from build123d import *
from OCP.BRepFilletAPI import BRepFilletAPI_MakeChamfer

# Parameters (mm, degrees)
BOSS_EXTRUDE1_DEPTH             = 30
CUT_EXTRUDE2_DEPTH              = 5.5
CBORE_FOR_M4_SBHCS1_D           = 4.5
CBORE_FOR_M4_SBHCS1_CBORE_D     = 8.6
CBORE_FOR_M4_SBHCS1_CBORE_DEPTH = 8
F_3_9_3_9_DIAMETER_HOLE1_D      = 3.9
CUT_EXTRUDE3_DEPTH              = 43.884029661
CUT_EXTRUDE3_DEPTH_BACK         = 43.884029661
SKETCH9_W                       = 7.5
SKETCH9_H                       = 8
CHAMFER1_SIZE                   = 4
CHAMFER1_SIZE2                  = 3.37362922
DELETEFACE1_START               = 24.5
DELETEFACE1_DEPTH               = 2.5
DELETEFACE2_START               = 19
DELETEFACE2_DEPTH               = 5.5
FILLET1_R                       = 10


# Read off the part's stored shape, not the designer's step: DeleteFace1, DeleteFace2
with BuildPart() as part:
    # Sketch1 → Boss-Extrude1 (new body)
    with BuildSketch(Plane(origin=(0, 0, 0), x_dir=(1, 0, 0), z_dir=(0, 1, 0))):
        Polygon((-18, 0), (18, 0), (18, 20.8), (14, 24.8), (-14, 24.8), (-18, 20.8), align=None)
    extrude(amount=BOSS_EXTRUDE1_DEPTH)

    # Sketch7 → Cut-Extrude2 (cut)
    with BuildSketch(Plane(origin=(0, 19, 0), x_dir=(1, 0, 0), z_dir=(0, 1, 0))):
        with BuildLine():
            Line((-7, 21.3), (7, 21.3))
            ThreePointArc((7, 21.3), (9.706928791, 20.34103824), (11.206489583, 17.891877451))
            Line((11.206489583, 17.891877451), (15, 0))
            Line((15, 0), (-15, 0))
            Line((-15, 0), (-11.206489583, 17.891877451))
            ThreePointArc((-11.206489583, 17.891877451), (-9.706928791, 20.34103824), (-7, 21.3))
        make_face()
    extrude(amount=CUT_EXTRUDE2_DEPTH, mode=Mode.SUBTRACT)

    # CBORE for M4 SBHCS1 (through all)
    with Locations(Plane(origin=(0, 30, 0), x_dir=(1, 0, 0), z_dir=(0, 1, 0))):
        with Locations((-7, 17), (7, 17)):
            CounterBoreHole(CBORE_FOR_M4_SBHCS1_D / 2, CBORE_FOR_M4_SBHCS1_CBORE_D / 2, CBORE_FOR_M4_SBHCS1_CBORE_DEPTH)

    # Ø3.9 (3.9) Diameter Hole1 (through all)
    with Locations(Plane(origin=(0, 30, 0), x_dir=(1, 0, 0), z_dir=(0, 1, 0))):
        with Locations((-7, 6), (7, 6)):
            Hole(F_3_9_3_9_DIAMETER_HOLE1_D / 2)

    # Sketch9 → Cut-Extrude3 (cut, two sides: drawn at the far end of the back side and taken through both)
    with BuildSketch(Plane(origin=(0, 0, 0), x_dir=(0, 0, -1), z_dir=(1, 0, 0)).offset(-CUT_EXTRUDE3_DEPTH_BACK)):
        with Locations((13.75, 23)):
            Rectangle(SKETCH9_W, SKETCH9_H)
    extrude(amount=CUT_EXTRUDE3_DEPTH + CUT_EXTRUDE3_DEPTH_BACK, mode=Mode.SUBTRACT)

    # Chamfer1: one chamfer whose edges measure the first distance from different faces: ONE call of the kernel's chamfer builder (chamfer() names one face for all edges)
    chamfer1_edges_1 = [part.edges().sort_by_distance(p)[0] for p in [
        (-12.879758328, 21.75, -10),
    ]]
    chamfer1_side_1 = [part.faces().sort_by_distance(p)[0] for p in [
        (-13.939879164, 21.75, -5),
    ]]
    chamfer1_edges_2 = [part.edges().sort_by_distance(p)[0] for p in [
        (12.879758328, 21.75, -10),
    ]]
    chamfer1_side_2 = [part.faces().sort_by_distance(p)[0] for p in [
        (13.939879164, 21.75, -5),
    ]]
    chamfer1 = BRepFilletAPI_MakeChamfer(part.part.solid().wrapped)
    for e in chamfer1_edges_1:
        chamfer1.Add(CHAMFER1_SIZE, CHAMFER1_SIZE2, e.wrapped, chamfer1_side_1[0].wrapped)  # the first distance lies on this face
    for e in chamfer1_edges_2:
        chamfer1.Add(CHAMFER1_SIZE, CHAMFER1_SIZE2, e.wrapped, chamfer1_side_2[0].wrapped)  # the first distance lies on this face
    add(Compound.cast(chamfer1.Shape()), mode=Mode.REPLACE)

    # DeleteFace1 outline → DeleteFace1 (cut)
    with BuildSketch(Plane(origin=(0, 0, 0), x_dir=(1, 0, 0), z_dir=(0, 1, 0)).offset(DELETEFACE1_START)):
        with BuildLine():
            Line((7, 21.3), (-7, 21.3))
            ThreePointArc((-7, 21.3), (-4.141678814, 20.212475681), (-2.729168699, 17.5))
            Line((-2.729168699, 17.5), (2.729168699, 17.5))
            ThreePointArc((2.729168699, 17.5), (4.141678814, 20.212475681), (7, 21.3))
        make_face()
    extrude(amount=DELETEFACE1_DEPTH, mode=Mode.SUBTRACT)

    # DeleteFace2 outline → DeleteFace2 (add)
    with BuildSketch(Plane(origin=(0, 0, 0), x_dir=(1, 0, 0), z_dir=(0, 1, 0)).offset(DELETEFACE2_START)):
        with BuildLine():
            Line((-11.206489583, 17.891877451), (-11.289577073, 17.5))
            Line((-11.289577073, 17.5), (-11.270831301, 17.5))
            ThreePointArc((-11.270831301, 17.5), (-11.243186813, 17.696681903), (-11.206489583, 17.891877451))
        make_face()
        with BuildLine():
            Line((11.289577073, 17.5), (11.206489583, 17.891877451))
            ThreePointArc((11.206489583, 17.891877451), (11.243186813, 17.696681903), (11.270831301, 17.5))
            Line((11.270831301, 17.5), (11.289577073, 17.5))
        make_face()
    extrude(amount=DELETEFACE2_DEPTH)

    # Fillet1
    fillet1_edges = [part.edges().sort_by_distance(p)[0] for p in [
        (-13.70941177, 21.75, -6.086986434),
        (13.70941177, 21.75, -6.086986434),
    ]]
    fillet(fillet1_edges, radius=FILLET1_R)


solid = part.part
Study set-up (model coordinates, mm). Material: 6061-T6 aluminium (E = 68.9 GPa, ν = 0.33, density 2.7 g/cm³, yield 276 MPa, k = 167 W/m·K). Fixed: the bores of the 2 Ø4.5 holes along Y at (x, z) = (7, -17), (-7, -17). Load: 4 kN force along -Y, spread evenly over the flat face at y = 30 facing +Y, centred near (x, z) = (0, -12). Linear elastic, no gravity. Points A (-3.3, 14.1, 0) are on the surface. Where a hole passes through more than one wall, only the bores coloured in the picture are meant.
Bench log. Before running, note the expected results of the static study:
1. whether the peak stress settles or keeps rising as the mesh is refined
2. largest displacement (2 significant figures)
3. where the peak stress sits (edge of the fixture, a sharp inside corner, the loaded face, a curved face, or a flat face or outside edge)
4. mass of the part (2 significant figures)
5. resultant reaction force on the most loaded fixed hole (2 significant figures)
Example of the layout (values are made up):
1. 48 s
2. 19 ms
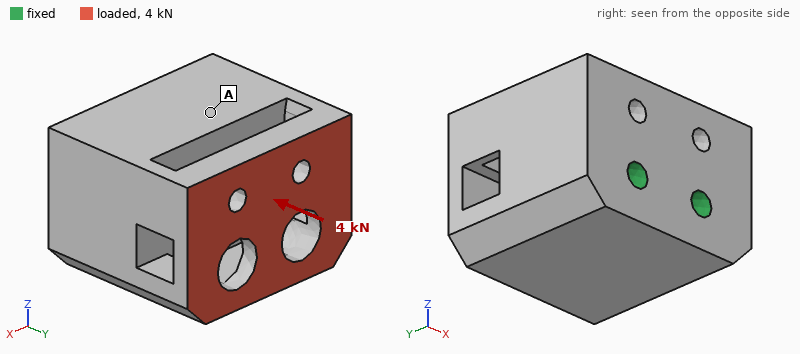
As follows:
1. keeps rising
2. 61 µm
3. a sharp inside corner
4. 55 g
5. 2.0 kN
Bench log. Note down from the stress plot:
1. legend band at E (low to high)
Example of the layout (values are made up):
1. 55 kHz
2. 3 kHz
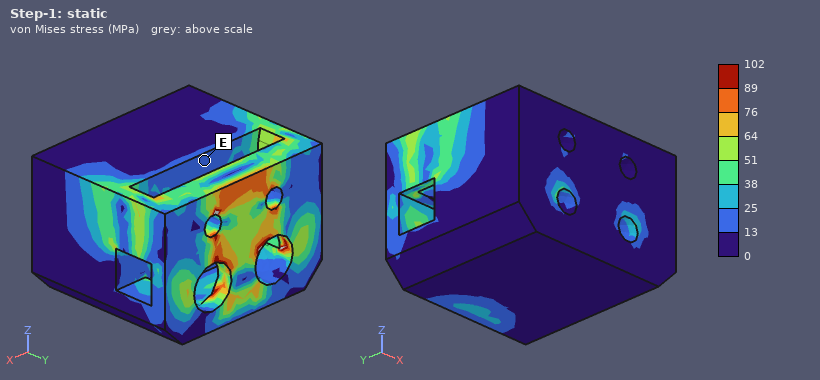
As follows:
1. 13 to 25 MPa
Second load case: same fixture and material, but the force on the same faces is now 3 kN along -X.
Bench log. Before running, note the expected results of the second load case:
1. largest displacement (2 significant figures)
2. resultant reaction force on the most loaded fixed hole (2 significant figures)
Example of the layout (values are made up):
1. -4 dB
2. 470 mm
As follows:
1. 44 µm
2. 2.4 kN
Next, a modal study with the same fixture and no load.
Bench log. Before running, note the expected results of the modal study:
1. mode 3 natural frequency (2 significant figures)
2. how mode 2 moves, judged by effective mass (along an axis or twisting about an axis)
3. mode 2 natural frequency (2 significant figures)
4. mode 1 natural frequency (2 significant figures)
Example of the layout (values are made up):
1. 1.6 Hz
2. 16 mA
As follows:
1. 17 kHz
2. along X
3. 15 kHz
4. 14 kHz
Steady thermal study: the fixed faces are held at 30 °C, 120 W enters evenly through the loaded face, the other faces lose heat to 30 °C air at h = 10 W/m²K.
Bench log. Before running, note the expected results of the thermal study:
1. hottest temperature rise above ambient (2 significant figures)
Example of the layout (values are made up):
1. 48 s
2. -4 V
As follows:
1. 75 K
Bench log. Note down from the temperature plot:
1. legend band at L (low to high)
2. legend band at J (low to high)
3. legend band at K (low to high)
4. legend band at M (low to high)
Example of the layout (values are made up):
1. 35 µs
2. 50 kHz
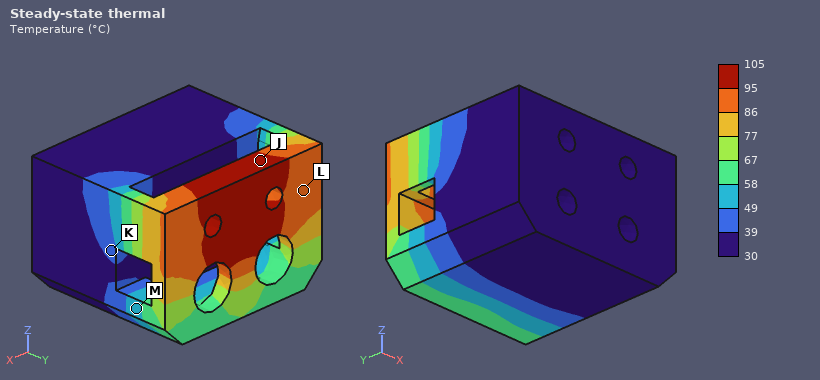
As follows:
1. 86 to 95 °C
2. 95 to 105 °C
3. 39 to 49 °C
4. 49 to 58 °C
